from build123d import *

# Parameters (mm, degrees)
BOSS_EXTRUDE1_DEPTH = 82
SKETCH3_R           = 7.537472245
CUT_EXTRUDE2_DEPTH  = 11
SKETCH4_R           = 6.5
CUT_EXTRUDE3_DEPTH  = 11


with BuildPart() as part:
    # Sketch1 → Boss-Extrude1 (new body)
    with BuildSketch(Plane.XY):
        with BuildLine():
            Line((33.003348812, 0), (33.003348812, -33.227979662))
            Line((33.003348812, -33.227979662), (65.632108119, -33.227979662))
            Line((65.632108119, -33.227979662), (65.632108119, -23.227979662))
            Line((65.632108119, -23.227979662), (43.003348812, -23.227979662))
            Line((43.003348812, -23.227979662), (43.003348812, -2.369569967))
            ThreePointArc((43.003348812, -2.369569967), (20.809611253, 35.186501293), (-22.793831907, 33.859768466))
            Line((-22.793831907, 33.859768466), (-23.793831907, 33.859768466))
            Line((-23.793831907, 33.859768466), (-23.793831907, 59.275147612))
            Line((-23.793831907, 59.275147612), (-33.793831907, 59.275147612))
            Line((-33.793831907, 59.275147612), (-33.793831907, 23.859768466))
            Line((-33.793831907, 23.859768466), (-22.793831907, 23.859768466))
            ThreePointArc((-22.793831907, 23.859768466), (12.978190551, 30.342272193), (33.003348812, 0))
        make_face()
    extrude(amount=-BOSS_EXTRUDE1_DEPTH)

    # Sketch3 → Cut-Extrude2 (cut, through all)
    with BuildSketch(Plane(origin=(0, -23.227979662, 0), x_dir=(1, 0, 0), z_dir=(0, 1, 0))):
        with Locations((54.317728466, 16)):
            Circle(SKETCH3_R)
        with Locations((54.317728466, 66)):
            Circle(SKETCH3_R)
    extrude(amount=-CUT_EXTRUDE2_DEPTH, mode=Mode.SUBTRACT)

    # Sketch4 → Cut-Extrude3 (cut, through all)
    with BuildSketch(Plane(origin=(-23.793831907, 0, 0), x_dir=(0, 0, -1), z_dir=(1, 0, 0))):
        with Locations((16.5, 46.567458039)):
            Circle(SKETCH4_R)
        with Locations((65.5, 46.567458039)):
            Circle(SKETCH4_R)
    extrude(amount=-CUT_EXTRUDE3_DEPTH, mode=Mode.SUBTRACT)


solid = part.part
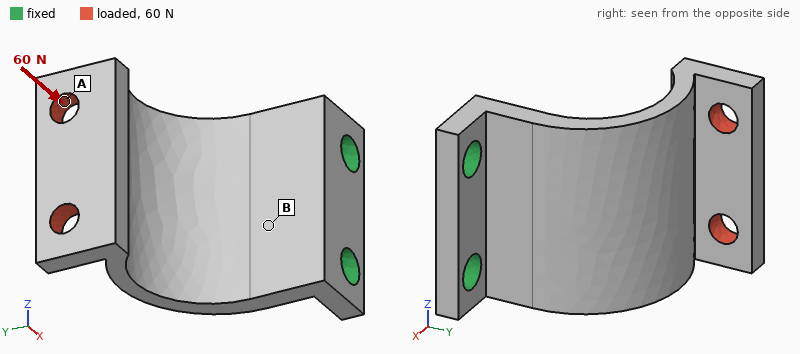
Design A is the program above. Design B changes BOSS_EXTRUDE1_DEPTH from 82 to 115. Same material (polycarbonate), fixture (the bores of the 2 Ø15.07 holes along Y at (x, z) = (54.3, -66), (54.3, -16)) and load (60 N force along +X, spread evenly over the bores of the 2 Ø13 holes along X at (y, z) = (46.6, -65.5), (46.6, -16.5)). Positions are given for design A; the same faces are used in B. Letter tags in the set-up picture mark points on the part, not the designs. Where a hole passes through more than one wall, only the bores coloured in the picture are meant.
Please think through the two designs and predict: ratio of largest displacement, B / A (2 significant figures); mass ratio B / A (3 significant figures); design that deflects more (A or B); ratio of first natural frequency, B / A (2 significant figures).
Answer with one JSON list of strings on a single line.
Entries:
["0.80", "1.42", "A", "0.96"]
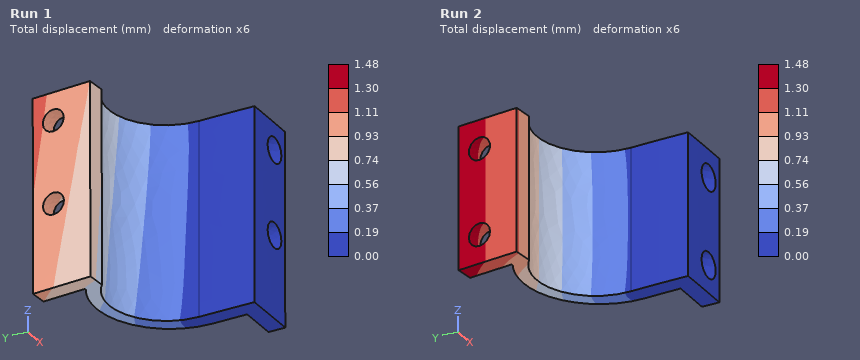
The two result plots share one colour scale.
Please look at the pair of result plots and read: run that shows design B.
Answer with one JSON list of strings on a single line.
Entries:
["Run 1"]
